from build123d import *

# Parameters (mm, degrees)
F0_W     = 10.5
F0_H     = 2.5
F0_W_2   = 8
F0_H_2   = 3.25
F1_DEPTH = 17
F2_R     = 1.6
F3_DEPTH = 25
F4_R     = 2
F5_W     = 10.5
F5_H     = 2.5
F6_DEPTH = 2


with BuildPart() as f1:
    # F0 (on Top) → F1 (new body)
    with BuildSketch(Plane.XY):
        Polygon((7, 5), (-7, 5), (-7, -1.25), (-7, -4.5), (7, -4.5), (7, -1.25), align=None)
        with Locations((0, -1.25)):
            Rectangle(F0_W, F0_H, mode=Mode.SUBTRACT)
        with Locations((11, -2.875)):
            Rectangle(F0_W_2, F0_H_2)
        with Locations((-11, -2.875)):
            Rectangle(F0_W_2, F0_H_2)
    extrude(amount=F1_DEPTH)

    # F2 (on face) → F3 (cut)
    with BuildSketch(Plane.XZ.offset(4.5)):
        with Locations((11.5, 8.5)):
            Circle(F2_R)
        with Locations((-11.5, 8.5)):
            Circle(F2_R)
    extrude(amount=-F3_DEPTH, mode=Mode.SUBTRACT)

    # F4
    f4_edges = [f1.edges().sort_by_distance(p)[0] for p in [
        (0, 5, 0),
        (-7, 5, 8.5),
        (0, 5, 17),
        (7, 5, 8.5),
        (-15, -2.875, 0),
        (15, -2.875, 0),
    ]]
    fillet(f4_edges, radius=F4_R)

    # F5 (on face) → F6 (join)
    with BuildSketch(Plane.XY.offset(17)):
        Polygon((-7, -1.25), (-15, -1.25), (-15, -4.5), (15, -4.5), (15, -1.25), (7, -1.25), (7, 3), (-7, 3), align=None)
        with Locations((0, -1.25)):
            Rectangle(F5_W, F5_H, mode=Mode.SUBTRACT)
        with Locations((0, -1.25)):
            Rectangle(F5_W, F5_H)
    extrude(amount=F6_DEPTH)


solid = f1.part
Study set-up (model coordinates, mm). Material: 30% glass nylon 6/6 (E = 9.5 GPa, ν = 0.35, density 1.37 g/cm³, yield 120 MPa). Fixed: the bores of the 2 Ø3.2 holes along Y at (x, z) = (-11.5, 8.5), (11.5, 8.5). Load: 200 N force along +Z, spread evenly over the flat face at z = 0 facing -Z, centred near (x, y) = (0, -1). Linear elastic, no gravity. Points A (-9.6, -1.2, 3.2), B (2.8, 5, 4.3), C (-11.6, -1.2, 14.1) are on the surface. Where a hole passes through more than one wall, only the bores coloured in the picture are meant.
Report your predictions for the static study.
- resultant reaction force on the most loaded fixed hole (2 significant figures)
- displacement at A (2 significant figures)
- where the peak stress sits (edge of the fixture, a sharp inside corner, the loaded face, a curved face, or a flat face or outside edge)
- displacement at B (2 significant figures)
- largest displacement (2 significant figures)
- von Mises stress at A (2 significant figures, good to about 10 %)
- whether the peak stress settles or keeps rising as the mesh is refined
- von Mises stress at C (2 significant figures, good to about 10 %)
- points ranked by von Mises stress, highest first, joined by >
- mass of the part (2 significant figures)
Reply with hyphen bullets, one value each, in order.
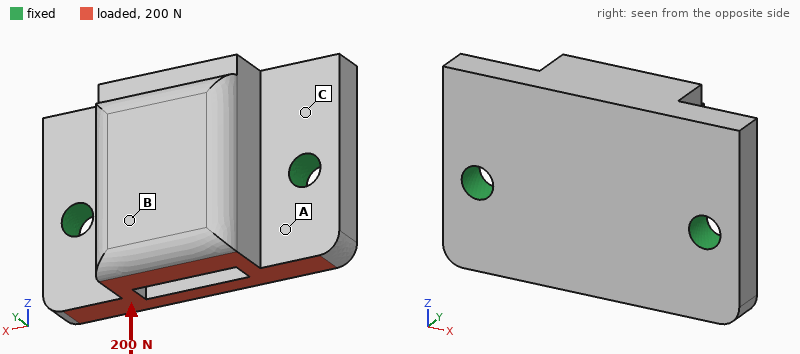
- 100 N
- 5.2 µm
- edge of the fixture
- 14 µm
- 17 µm
- 4.2 MPa
- keeps rising
- 2.7 MPa
- A > C > B
- 4.0 g
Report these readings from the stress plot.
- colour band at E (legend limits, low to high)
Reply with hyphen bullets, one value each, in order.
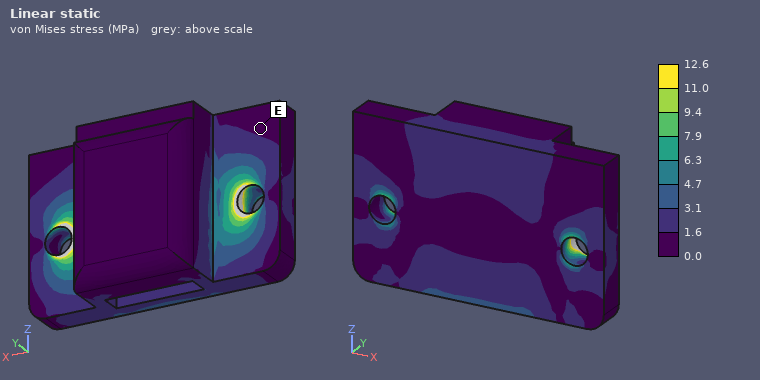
- 0.0 to 1.6 MPa
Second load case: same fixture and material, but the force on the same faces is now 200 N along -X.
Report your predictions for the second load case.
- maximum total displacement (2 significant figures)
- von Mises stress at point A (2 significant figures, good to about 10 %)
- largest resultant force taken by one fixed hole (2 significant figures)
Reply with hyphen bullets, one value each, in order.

- 12 µm
- 5.0 MPa
- 120 N
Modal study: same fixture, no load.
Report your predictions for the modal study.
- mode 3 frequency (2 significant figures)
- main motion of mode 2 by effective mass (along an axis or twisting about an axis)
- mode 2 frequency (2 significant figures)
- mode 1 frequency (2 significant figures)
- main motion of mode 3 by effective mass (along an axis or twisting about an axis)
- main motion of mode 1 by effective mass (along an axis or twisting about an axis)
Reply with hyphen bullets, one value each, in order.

- 17 kHz
- along Y
- 12 kHz
- 6600 Hz
- along X
- along Z
